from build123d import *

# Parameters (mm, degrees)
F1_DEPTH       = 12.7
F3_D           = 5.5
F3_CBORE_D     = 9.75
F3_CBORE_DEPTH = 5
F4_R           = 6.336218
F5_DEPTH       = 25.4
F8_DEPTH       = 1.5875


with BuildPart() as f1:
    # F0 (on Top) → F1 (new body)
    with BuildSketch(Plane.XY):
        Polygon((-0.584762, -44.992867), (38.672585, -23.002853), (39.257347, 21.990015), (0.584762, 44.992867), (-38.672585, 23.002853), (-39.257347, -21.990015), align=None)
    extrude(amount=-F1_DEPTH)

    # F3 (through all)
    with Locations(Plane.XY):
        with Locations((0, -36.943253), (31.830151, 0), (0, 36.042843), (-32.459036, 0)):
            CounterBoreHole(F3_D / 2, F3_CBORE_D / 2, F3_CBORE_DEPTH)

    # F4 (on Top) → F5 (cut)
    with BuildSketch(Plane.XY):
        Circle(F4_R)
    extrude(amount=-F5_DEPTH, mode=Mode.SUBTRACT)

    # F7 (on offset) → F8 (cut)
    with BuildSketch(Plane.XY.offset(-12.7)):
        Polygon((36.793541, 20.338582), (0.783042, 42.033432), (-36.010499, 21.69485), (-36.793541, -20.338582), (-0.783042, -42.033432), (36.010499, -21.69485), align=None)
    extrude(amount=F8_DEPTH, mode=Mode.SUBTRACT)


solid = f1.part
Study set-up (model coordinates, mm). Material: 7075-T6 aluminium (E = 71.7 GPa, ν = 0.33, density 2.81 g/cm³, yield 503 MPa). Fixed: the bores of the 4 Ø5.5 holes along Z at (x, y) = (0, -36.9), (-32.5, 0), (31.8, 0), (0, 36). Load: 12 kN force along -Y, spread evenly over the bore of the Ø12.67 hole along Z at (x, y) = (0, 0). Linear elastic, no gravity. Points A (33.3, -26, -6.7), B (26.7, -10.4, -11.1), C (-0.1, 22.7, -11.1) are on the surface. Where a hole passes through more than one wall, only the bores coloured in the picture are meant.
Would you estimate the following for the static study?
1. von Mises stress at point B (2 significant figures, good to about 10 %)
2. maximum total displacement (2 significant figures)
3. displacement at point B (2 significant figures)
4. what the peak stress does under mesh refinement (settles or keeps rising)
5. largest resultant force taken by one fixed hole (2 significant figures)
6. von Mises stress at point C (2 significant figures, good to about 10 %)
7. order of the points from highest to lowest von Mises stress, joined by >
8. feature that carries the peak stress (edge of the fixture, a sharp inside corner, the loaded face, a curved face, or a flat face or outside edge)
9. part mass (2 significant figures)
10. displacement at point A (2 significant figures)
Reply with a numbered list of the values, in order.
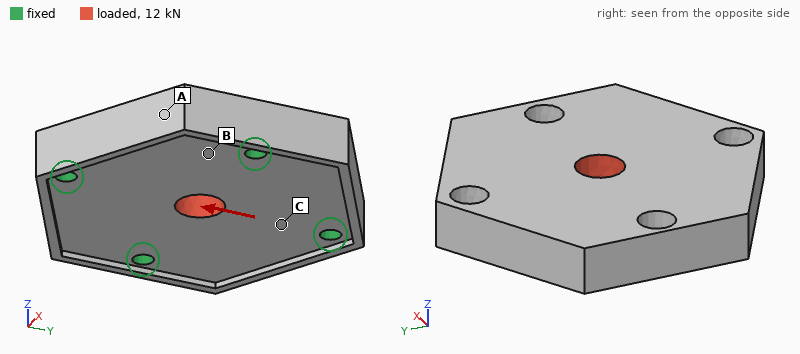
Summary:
1. 13 MPa
2. 11 µm
3. 2.8 µm
4. keeps rising
5. 3.6 kN
6. 27 MPa
7. C > B > A
8. edge of the fixture
9. 160 g
10. 3.9 µm
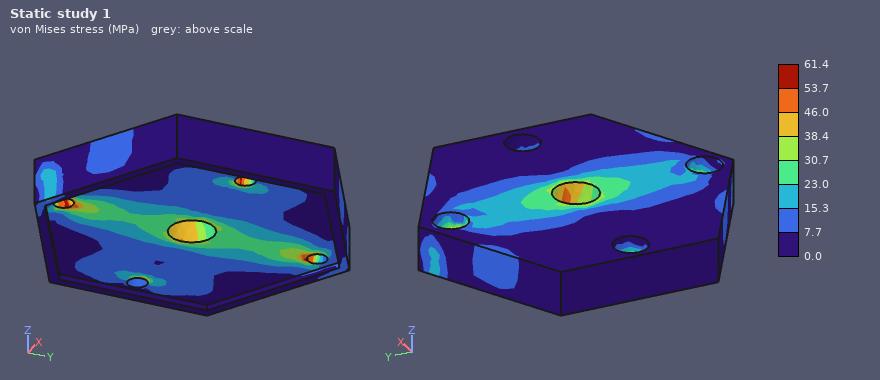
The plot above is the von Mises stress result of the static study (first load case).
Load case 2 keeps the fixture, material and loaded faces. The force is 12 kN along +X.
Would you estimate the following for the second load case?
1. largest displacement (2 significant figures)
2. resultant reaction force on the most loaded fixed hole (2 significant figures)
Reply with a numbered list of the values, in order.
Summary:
1. 11 µm
2. 4.1 kN
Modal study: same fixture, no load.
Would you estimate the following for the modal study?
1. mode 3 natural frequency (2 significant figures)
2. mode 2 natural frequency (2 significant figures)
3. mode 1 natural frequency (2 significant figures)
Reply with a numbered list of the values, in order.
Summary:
1. 12 kHz
2. 12 kHz
3. 11 kHz
